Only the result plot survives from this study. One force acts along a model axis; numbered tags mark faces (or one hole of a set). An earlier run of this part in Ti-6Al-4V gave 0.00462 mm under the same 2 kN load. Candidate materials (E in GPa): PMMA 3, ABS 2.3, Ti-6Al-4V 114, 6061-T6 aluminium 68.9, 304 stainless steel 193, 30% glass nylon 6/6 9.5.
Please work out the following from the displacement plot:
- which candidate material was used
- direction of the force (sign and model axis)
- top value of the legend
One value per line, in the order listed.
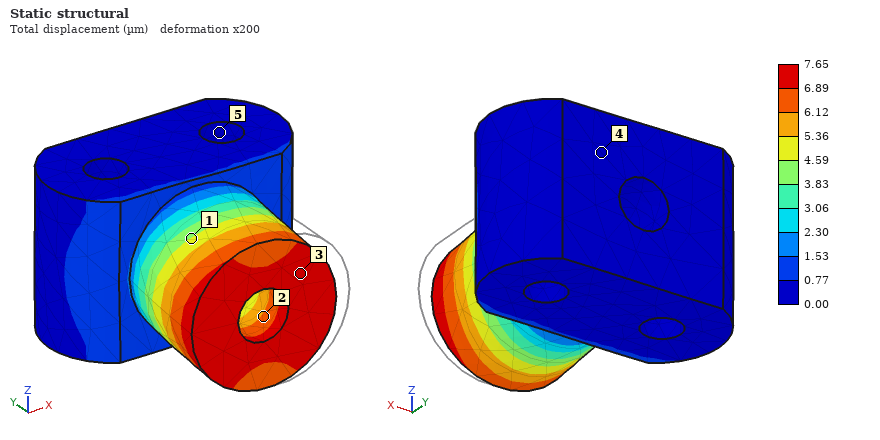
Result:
6061-T6 aluminium
-X
7.65 µm
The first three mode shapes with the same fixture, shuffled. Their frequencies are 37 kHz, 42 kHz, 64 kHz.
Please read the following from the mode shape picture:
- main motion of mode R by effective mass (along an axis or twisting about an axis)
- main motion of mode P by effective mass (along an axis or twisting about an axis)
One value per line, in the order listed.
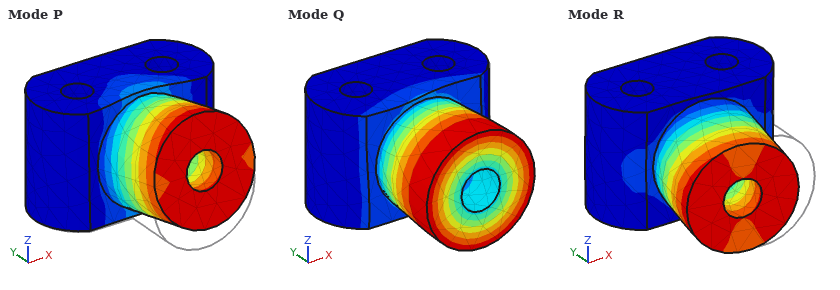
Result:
along X
along Z
